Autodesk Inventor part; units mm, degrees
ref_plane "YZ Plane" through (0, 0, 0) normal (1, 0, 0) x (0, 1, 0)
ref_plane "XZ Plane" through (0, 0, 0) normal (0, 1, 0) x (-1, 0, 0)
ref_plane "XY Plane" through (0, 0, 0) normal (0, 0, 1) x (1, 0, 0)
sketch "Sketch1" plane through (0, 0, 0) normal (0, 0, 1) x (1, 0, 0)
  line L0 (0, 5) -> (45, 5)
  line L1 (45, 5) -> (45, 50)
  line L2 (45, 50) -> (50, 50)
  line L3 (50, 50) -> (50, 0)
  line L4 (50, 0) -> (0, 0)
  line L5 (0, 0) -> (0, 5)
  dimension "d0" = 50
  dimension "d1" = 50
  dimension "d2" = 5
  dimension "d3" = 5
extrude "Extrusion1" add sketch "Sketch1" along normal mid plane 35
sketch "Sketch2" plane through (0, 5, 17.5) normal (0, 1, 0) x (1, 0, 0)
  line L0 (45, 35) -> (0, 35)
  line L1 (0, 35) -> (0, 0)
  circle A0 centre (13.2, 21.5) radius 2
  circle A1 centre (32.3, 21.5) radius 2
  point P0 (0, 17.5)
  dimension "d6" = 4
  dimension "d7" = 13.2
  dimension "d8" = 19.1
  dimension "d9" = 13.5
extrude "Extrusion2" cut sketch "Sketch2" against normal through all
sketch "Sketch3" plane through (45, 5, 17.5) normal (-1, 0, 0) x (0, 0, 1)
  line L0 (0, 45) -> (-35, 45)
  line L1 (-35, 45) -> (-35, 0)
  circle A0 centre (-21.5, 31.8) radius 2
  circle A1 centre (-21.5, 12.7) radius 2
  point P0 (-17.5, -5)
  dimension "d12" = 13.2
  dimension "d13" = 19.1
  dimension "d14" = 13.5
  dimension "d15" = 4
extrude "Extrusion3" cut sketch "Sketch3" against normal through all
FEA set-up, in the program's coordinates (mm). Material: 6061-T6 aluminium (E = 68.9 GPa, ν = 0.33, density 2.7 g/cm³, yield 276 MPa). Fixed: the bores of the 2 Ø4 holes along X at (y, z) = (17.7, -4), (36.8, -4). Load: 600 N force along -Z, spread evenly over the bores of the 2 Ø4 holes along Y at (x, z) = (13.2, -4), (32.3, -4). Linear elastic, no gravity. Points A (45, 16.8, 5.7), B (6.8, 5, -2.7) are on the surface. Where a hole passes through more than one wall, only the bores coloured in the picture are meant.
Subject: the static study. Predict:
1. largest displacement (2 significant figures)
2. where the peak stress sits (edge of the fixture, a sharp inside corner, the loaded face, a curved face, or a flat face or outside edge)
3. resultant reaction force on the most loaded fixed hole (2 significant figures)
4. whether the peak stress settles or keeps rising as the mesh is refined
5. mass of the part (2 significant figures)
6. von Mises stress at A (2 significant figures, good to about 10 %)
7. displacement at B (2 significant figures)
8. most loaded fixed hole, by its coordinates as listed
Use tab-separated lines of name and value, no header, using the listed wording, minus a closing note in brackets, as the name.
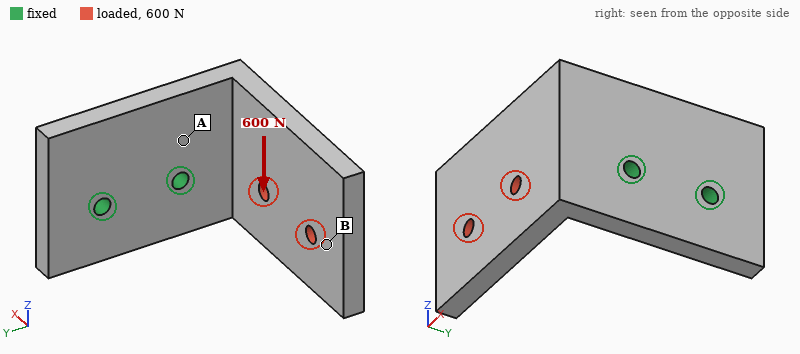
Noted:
largest displacement	0.33 mm
where the peak stress sits	edge of the fixture
resultant reaction force on the most loaded fixed hole	980 N
whether the peak stress settles or keeps rising as the mesh is refined	keeps rising
mass of the part	44 g
von Mises stress at A	51 MPa
displacement at B	0.26 mm
most loaded fixed hole, by its coordinates as listed	(17.7, -4)
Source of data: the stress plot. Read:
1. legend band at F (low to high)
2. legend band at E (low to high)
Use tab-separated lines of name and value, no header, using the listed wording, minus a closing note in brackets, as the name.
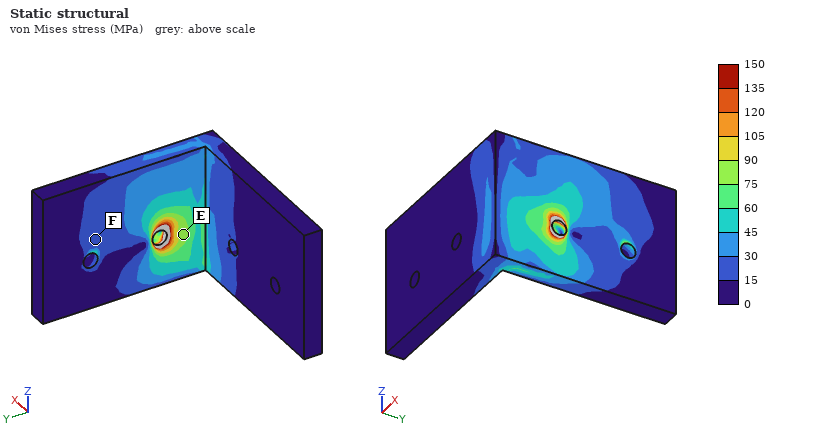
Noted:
legend band at F	15 to 30 MPa
legend band at E	75 to 90 MPa
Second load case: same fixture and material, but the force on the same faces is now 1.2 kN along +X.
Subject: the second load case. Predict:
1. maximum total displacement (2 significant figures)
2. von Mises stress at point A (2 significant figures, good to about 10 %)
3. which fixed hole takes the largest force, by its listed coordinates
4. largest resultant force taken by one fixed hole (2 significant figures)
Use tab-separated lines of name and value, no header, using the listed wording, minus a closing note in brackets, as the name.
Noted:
maximum total displacement	0.33 mm
von Mises stress at point A	59 MPa
which fixed hole takes the largest force, by its listed coordinates	(17.7, -4)
largest resultant force taken by one fixed hole	1.6 kN
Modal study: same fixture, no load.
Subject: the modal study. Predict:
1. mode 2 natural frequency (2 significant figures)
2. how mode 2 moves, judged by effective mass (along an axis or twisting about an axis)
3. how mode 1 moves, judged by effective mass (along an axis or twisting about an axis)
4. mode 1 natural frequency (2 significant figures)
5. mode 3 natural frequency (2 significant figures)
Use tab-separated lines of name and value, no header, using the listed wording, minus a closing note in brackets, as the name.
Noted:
mode 2 natural frequency	1800 Hz
how mode 2 moves, judged by effective mass	along Z
how mode 1 moves, judged by effective mass	along Y
mode 1 natural frequency	1200 Hz
mode 3 natural frequency	4800 Hz
